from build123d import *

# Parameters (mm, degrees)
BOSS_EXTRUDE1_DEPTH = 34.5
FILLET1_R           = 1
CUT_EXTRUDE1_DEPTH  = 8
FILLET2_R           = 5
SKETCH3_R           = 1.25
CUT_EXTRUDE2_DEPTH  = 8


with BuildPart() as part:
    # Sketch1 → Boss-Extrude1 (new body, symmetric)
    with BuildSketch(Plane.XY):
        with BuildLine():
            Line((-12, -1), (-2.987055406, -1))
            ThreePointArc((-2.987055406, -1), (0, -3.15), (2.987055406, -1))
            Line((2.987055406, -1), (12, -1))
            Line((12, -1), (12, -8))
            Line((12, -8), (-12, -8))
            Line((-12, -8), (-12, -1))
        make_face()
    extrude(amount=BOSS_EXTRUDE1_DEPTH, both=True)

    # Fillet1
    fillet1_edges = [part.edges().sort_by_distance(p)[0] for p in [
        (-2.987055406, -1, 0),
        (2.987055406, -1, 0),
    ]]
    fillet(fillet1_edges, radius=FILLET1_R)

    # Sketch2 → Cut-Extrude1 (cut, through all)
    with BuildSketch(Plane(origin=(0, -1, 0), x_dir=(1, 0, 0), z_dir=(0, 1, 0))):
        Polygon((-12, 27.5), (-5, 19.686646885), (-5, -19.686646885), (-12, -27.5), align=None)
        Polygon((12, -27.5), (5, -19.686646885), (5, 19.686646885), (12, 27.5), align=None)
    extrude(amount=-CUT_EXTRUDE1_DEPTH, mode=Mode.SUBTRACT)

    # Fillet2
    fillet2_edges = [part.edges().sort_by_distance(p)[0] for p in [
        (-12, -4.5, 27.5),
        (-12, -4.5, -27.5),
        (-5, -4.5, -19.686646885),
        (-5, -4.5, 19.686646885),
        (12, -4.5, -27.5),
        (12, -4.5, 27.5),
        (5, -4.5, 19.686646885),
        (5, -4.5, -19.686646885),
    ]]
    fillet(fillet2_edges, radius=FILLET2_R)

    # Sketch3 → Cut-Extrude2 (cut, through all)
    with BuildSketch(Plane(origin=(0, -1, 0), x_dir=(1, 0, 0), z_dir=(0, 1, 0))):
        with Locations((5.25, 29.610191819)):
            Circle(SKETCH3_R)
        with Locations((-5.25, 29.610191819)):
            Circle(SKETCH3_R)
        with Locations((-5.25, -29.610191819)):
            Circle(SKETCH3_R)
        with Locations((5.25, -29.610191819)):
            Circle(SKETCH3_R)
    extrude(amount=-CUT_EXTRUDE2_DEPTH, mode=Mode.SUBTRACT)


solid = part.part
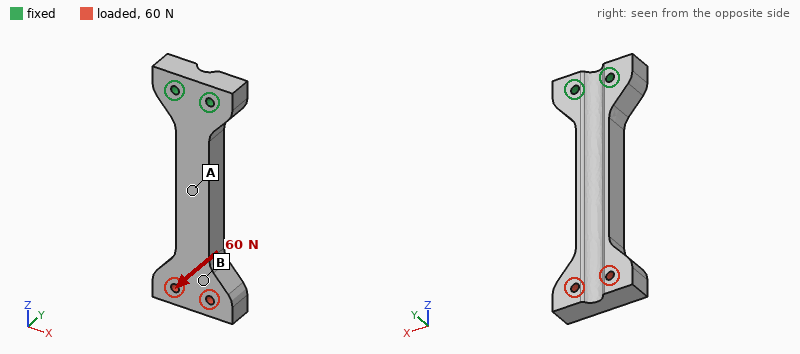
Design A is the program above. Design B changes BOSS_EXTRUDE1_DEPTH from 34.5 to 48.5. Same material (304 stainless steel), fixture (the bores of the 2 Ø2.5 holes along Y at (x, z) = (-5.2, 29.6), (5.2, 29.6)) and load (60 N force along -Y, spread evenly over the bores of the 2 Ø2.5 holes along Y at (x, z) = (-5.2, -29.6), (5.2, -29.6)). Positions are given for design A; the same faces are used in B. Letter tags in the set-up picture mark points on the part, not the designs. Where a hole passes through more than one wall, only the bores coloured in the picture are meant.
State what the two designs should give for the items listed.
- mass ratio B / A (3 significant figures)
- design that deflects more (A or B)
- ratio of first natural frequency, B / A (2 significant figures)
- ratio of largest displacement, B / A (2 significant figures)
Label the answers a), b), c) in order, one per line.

a) 1.72
b) B
c) 0.59
d) 1.3
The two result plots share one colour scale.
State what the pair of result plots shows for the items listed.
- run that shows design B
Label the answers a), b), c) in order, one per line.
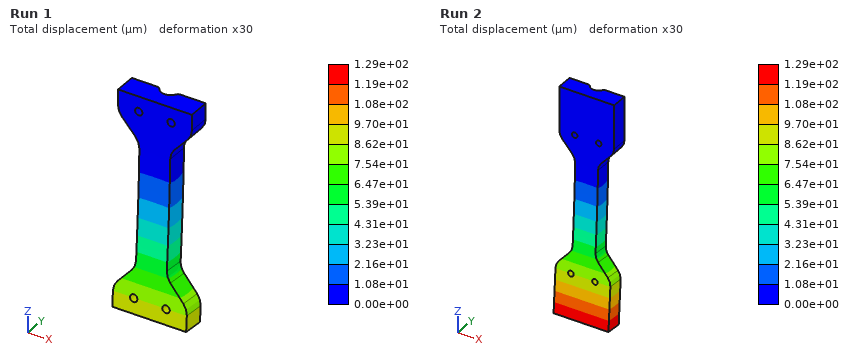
a) Run 2
